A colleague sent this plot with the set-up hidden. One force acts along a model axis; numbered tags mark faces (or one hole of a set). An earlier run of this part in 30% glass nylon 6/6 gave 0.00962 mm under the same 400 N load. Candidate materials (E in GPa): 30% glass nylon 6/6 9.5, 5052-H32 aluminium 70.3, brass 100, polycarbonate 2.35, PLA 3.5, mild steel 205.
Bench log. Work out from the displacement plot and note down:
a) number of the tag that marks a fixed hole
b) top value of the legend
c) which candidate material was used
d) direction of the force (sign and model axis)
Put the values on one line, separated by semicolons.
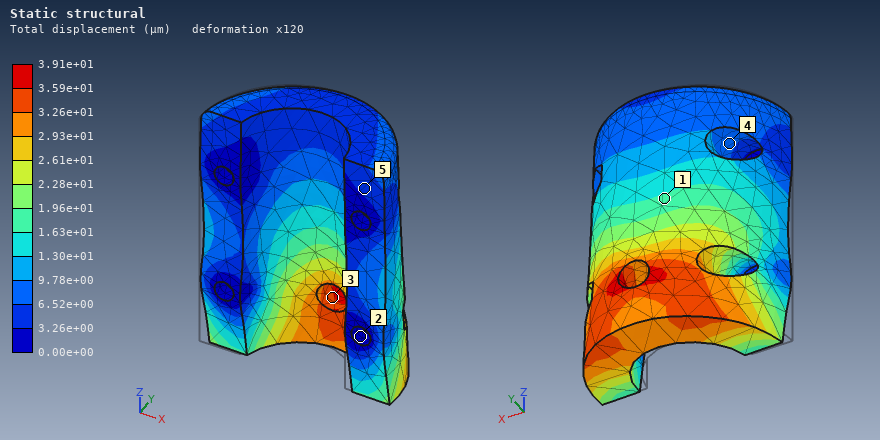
2; 3.91e+01 µm; polycarbonate; +X
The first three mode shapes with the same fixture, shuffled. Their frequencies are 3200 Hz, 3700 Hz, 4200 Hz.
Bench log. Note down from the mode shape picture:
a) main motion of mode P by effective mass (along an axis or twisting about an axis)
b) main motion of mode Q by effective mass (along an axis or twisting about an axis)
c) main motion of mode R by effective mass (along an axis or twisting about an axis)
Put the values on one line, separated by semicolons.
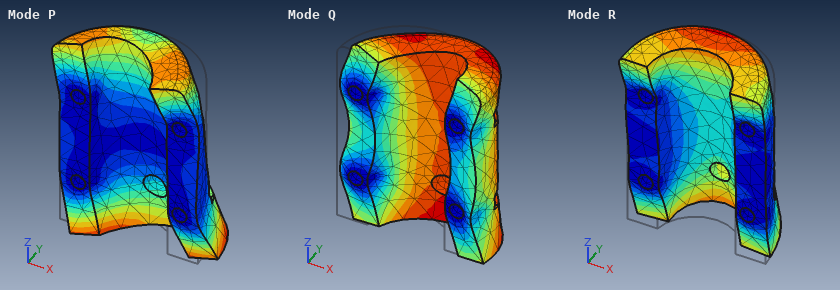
twisting about Y; along X; along Z
